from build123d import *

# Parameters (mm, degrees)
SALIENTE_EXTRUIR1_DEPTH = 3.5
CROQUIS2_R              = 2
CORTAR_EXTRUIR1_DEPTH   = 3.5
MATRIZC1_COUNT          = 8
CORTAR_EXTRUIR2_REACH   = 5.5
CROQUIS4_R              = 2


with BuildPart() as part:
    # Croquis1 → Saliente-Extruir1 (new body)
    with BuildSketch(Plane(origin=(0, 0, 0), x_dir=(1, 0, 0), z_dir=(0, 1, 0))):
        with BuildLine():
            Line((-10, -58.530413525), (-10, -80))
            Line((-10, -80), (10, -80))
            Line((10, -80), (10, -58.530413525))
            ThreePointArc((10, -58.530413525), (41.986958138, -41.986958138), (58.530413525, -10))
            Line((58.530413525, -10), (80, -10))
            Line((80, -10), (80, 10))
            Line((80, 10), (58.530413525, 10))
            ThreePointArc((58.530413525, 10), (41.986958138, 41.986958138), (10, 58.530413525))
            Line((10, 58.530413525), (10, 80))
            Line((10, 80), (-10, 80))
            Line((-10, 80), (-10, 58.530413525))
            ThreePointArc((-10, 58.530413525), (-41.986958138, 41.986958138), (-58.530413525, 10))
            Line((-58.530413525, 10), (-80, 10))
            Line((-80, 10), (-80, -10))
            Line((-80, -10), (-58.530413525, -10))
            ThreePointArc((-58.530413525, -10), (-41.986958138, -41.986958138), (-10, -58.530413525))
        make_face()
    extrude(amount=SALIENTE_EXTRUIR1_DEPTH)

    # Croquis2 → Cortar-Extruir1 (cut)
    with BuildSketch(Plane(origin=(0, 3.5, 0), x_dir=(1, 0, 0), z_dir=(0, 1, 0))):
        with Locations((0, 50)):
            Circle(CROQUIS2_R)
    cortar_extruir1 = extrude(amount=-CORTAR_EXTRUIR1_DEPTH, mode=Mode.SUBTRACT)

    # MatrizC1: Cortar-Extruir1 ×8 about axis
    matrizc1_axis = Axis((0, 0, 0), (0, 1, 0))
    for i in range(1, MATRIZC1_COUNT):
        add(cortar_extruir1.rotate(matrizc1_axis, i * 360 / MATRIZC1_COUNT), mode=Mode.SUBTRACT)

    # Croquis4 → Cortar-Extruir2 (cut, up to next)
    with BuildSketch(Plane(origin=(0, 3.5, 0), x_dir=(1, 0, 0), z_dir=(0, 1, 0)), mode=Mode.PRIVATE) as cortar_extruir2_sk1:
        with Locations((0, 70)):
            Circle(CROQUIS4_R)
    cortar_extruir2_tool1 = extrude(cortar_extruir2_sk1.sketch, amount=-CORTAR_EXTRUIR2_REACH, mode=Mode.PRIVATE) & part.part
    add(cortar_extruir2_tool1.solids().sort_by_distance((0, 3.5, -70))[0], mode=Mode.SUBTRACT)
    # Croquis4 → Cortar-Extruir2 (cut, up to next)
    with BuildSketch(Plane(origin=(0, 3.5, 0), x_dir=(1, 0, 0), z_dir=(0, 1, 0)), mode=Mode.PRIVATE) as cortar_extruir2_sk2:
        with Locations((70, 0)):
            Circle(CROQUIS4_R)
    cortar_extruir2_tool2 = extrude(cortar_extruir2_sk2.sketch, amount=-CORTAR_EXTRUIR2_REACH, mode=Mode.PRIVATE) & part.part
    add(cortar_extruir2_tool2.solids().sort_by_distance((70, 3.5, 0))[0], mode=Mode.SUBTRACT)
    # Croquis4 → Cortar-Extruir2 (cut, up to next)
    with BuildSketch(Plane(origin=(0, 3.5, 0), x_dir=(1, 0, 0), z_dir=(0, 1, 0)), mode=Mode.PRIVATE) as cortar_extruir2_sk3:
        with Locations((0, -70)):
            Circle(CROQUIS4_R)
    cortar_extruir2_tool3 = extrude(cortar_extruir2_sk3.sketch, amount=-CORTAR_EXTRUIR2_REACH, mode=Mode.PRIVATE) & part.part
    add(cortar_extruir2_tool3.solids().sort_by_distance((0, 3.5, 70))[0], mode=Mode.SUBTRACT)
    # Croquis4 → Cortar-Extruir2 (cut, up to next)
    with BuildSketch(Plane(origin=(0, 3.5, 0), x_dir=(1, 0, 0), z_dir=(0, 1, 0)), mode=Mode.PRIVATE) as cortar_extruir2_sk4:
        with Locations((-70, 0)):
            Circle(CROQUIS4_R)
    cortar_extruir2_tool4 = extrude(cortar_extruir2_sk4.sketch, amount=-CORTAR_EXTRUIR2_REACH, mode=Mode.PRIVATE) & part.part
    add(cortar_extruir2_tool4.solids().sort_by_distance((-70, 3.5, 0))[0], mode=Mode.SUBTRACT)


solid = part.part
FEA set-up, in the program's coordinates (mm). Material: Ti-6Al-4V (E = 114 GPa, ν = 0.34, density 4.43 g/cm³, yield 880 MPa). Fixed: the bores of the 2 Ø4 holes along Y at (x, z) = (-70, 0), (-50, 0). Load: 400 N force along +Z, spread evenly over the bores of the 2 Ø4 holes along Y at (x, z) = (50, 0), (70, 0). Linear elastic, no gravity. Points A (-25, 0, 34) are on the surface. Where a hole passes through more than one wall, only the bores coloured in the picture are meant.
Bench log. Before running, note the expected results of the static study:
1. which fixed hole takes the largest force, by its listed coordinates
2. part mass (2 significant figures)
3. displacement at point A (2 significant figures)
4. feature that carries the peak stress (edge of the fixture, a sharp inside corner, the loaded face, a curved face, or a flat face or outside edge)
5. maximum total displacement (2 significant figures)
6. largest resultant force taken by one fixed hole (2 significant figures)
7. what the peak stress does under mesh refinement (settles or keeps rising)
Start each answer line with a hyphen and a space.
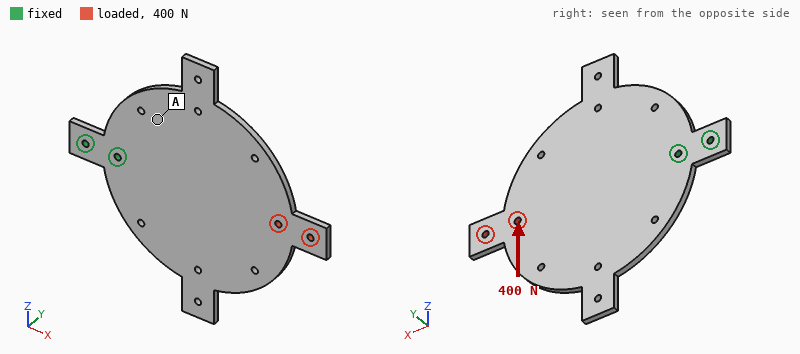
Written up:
- (-50, 0)
- 200 g
- 0.062 mm
- edge of the fixture
- 0.20 mm
- 2.2 kN
- keeps rising
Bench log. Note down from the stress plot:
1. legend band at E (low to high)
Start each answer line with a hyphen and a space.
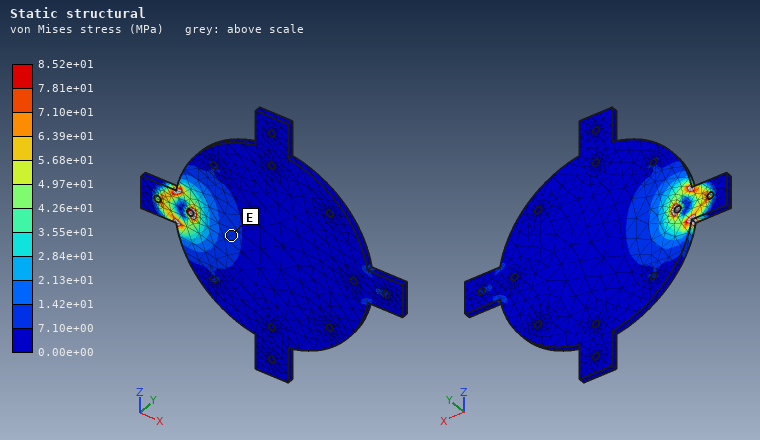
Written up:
- 7.10e+00 to 1.42e+01 MPa
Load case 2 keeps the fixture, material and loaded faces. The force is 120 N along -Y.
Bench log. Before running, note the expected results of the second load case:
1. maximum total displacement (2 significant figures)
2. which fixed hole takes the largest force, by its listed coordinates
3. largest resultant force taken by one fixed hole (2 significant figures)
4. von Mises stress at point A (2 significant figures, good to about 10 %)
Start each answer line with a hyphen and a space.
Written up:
- 2.4 mm
- (-50, 0)
- 410 N
- 41 MPa
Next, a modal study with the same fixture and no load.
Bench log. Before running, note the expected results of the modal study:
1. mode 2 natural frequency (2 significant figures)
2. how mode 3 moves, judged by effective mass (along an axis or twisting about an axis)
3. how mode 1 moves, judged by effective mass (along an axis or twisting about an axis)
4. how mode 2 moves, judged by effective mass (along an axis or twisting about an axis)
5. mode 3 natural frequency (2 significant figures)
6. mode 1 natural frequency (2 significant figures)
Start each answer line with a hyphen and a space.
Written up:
- 310 Hz
- along Y
- along Y
- twisting about X
- 750 Hz
- 190 Hz
